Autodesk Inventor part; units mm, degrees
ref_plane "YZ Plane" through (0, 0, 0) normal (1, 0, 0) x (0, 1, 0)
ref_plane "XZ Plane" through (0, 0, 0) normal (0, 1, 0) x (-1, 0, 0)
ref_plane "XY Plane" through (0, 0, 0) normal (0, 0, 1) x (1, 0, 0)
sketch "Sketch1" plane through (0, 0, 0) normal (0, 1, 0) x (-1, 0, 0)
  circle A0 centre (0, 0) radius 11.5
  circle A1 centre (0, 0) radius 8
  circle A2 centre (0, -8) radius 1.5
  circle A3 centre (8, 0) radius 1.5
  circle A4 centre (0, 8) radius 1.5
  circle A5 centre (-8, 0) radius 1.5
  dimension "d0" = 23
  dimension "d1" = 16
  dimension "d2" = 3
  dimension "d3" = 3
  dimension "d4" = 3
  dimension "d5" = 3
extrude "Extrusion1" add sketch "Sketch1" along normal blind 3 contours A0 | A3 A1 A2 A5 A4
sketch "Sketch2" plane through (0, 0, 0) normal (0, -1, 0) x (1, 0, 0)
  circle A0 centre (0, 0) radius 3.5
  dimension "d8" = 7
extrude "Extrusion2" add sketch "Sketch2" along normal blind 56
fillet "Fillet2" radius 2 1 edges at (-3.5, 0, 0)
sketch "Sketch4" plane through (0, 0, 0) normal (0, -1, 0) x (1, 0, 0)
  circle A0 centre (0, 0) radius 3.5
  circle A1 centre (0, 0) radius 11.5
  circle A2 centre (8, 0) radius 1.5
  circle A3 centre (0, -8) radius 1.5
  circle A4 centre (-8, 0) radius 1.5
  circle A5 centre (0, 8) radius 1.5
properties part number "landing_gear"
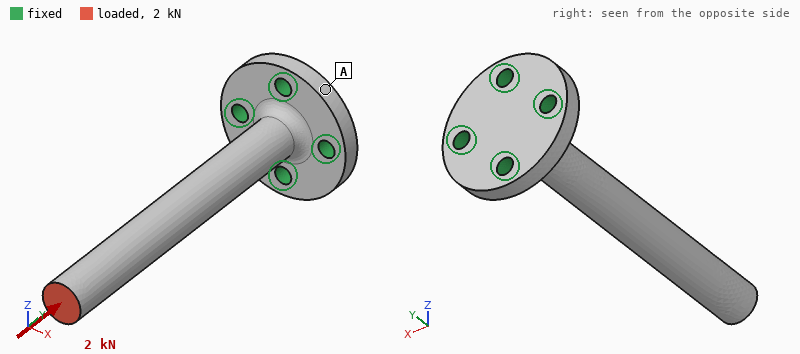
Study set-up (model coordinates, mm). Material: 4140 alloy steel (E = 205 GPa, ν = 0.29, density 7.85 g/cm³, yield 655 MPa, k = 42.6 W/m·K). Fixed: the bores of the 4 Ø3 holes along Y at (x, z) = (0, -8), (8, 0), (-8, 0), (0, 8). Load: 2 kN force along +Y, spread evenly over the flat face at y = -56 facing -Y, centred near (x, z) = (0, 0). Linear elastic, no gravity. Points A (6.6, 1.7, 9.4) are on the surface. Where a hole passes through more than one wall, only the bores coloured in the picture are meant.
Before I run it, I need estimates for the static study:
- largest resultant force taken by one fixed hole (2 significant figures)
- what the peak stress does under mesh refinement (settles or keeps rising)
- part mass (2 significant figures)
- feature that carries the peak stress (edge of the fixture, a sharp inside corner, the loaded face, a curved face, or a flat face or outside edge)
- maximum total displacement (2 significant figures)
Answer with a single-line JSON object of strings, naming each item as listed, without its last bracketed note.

{"largest resultant force taken by one fixed hole": "530 N", "what the peak stress does under mesh refinement": "keeps rising", "part mass": "26 g", "feature that carries the peak stress": "edge of the fixture", "maximum total displacement": "16 µm"}
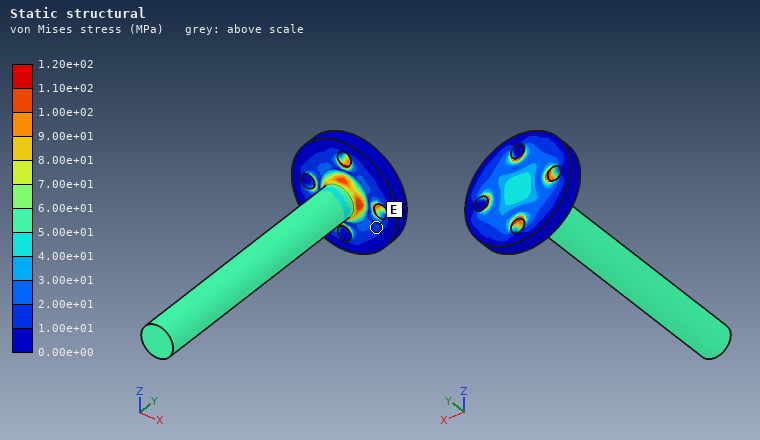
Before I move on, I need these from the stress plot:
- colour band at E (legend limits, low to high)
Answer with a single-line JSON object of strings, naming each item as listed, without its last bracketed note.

{"colour band at E": "1.00e+01 to 2.00e+01 MPa"}
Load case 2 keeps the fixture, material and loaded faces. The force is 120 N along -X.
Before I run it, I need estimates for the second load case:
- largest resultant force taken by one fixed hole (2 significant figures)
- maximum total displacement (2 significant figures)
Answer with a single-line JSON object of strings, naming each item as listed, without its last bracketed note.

{"largest resultant force taken by one fixed hole": "500 N", "maximum total displacement": "0.31 mm"}
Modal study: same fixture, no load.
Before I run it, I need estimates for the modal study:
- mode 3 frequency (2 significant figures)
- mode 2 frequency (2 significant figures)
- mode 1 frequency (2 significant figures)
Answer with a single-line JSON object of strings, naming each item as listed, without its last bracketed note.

{"mode 3 frequency": "9100 Hz", "mode 2 frequency": "1500 Hz", "mode 1 frequency": "1500 Hz"}
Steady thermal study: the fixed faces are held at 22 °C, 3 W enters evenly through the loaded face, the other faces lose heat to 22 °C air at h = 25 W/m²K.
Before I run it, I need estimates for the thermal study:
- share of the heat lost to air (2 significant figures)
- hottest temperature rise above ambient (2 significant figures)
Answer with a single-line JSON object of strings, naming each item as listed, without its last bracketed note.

{"share of the heat lost to air": "39 %", "hottest temperature rise above ambient": "79 K"}
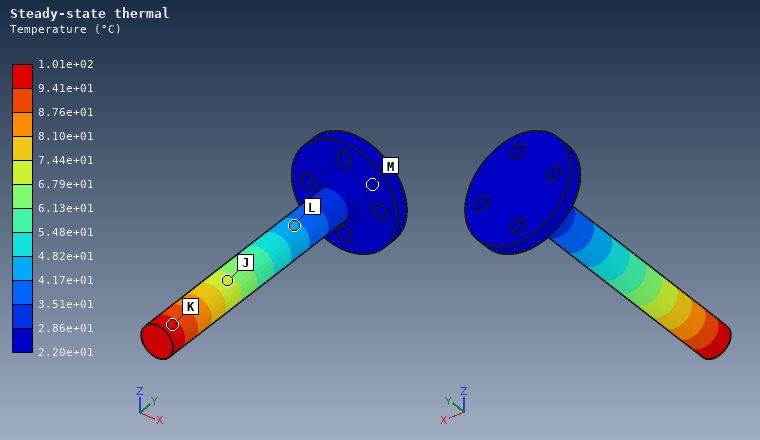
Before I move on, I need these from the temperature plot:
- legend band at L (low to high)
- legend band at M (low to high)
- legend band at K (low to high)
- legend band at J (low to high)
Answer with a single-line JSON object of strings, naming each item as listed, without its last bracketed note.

{"legend band at L": "4.17e+01 to 4.82e+01 °C", "legend band at M": "2.20e+01 to 2.86e+01 °C", "legend band at K": "9.41e+01 to 1.01e+02 °C", "legend band at J": "6.79e+01 to 7.44e+01 °C"}
